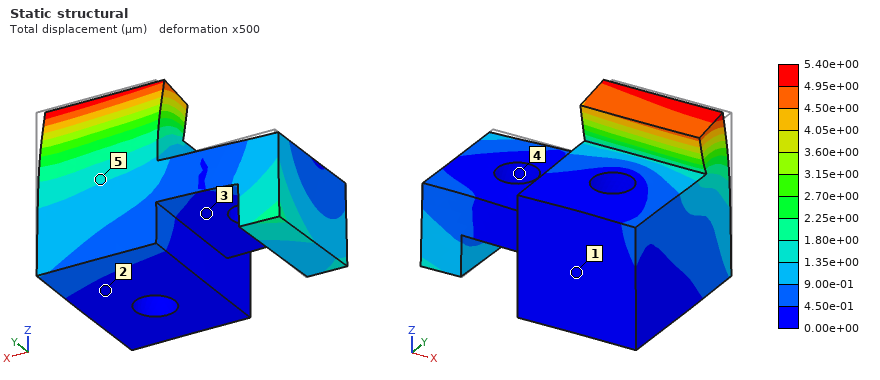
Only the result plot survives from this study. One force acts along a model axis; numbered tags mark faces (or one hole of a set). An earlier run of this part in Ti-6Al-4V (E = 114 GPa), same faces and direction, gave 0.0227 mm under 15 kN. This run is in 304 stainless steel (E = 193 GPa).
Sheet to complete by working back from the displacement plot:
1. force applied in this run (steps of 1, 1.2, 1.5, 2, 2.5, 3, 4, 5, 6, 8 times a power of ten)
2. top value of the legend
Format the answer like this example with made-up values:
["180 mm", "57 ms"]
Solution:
["6 kN", "5.40e+00 µm"]
